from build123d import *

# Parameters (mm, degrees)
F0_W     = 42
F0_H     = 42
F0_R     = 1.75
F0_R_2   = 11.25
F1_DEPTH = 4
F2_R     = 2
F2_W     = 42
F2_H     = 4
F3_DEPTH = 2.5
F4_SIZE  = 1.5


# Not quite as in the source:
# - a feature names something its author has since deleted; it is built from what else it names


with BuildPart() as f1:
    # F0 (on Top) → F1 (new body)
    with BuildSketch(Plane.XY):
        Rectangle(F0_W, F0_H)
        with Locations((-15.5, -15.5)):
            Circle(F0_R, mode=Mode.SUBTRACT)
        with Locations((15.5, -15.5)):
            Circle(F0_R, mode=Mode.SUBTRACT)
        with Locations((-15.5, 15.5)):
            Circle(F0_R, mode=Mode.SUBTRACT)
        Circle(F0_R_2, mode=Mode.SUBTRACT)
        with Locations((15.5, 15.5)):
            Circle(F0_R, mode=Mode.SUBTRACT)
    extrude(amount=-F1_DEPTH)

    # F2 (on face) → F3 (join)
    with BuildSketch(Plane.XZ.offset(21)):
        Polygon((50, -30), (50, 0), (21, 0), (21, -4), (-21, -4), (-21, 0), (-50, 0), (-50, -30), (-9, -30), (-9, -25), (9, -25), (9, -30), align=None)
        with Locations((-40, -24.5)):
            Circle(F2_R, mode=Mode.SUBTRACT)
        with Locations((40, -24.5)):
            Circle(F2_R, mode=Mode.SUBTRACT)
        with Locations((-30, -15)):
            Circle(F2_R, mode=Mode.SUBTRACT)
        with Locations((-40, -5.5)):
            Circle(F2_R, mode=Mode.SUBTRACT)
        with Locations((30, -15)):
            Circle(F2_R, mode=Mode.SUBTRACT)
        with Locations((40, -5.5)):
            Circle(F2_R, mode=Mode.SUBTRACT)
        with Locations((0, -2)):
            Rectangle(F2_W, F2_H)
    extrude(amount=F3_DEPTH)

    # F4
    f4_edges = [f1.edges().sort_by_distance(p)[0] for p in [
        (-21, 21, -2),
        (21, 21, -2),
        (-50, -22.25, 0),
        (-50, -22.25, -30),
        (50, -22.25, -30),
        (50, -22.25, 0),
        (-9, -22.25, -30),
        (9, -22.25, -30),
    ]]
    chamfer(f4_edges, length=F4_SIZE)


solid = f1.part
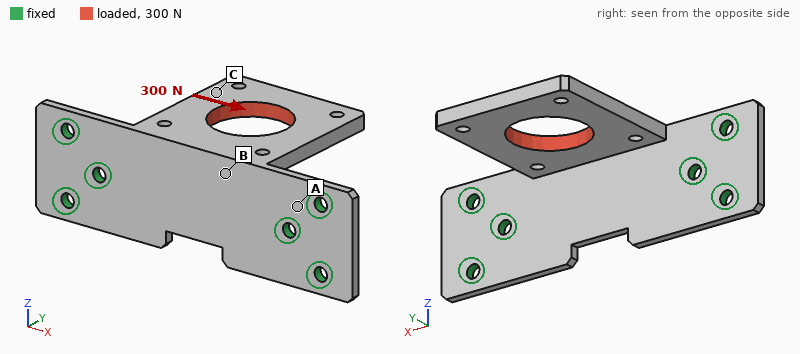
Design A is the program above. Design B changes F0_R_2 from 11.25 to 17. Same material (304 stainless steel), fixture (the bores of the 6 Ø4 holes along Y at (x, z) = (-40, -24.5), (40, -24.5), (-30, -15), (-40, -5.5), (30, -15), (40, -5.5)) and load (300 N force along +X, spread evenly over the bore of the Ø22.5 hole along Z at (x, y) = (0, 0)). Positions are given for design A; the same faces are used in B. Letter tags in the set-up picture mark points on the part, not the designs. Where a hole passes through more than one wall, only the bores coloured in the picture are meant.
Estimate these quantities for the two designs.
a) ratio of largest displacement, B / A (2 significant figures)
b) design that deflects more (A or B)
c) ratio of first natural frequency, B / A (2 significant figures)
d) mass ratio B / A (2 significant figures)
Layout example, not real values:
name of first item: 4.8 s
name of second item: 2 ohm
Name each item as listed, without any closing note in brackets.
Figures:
ratio of largest displacement, B / A: 1.4
design that deflects more: B
ratio of first natural frequency, B / A: 1.1
mass ratio B / A: 0.84
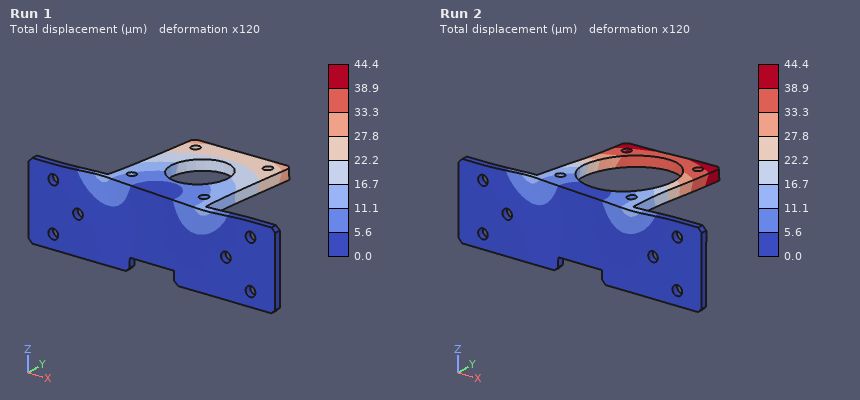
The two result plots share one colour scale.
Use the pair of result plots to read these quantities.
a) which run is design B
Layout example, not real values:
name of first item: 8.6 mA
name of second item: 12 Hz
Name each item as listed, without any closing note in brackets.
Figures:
which run is design B: Run 2
